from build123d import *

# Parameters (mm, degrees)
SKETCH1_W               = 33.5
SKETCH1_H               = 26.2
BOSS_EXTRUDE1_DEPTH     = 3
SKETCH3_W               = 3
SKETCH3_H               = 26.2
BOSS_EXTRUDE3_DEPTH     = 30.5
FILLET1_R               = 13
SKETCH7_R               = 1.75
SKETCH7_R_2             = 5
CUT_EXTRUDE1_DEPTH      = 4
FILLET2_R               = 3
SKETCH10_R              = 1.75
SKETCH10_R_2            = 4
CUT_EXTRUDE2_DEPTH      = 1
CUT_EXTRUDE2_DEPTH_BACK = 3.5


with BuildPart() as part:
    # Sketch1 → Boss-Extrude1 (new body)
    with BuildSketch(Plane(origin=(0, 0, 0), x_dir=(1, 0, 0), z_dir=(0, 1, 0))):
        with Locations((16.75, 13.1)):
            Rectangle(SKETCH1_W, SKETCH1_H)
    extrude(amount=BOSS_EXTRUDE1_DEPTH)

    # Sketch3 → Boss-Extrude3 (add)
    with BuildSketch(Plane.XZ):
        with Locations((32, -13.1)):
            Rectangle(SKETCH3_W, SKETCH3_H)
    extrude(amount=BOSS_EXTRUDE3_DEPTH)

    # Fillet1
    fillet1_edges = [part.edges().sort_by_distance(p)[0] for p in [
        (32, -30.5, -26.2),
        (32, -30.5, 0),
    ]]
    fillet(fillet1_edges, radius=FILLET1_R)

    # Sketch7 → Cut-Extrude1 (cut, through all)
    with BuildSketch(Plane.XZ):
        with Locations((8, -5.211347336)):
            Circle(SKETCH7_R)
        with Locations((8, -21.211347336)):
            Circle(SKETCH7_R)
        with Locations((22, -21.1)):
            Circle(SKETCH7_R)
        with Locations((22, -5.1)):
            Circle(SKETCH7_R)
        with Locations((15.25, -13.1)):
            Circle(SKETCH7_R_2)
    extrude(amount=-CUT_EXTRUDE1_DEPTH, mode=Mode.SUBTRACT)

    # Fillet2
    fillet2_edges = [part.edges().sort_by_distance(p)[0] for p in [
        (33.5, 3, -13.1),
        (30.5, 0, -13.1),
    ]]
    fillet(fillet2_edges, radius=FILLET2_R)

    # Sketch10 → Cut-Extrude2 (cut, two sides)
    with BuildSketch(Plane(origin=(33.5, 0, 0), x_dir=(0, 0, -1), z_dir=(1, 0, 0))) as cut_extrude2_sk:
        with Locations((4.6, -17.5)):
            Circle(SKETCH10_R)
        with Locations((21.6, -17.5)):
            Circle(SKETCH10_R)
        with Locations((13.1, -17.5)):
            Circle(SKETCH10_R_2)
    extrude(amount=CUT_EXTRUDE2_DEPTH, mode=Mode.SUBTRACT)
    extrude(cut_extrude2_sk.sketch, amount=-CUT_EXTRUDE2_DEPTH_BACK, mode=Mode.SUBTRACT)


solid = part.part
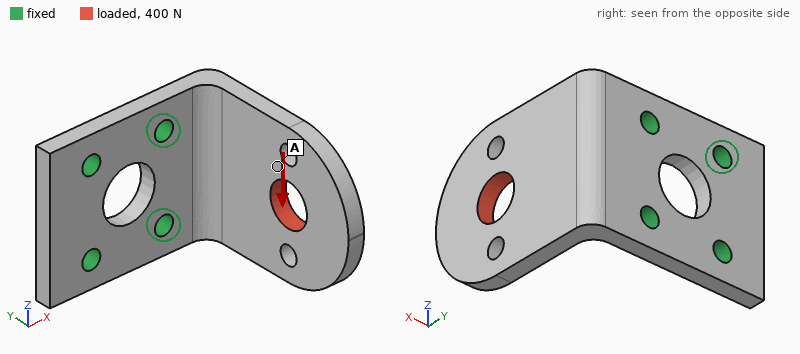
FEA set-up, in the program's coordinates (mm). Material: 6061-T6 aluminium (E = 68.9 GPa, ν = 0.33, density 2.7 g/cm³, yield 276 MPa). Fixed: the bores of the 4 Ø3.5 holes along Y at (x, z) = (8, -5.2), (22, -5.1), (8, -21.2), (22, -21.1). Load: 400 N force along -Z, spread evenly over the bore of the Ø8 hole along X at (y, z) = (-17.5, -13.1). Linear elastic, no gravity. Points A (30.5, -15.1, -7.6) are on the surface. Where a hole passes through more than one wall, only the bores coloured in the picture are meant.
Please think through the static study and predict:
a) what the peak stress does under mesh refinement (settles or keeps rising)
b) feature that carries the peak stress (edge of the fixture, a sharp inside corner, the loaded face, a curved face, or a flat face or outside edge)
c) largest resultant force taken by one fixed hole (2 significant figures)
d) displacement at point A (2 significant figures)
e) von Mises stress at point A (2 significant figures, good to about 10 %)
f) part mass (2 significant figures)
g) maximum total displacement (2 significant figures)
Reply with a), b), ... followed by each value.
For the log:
a) keeps rising
b) edge of the fixture
c) 510 N
d) 0.062 mm
e) 14 MPa
f) 11 g
g) 0.11 mm
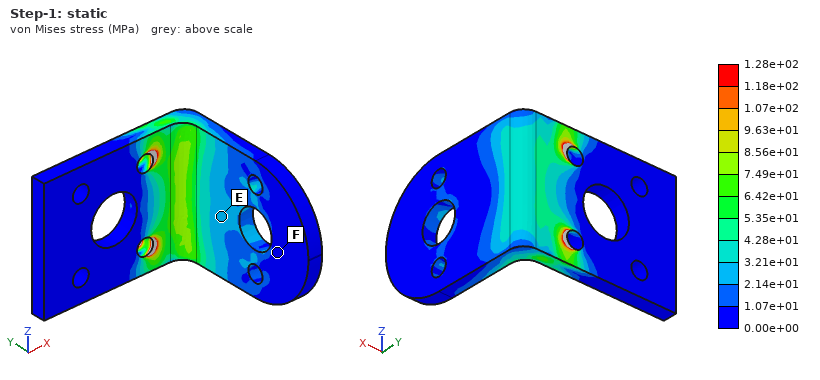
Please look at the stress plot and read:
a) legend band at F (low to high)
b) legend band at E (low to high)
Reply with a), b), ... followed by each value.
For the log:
a) 0.00e+00 to 1.07e+01 MPa
b) 2.14e+01 to 3.21e+01 MPa
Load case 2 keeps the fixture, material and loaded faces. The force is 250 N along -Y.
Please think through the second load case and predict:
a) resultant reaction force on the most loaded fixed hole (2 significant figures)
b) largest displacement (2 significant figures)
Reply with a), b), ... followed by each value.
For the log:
a) 130 N
b) 87 µm
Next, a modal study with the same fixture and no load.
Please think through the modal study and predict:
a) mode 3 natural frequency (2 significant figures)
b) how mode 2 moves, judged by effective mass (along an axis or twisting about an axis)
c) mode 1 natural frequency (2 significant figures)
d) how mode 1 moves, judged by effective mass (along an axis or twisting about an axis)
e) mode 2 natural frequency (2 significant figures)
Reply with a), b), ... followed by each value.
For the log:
a) 8400 Hz
b) along Z
c) 2200 Hz
d) along X
e) 5200 Hz
